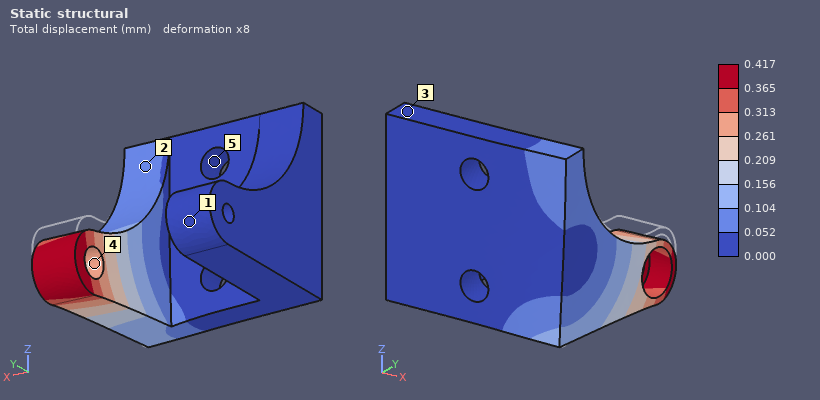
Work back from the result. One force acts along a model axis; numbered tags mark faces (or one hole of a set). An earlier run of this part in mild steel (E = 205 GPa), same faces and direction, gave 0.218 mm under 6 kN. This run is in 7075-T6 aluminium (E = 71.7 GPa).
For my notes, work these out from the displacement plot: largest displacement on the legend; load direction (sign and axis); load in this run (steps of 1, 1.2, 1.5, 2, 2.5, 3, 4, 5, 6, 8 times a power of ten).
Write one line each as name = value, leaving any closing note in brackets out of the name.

largest displacement on the legend = 0.417 mm
load direction = -Z
load in this run = 4 kN
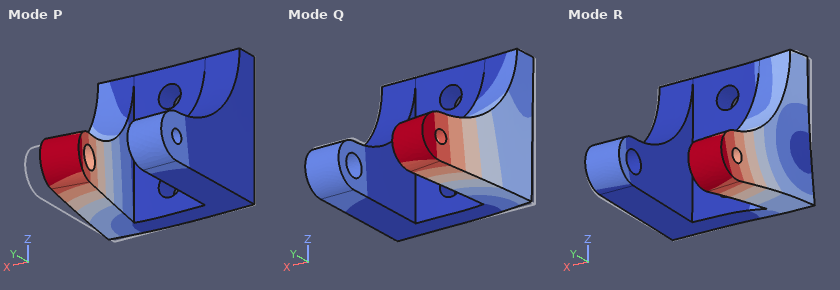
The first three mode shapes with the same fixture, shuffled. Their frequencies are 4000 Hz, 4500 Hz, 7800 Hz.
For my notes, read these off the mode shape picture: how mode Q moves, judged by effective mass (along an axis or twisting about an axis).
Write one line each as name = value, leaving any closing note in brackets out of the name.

how mode Q moves, judged by effective mass = along X
